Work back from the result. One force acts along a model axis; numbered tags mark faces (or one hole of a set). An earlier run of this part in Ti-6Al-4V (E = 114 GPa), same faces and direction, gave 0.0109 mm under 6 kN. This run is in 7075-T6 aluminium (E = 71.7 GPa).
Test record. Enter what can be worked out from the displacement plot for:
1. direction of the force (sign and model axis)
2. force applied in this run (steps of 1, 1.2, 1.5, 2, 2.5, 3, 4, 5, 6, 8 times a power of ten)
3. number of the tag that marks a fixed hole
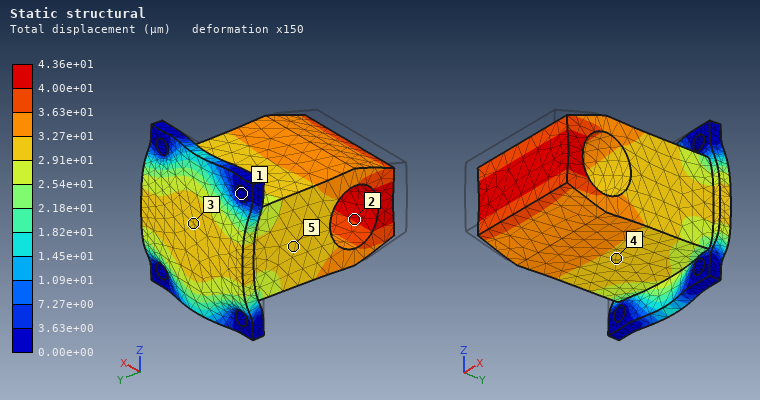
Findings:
+Y
15 kN
1
